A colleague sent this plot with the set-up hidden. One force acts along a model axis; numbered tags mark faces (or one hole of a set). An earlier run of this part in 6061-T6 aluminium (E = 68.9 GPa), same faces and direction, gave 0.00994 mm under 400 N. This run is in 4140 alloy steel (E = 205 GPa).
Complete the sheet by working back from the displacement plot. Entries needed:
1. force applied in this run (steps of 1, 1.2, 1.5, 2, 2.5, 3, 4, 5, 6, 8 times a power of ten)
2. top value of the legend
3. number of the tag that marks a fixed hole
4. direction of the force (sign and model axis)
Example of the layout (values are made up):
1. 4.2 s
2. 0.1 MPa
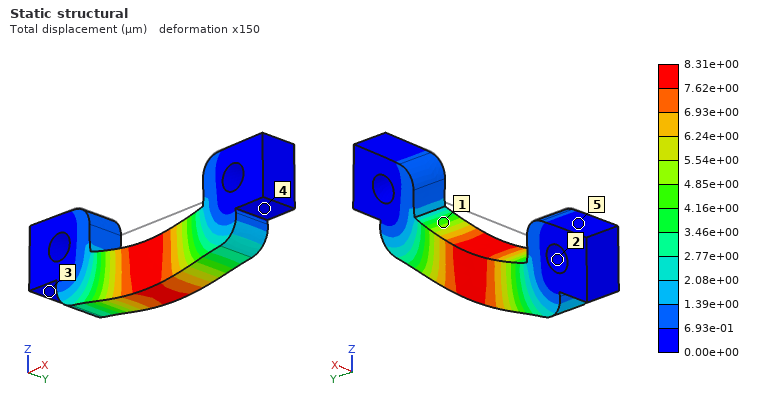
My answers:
1. 1 kN
2. 8.31e+00 µm
3. 2
4. -Z
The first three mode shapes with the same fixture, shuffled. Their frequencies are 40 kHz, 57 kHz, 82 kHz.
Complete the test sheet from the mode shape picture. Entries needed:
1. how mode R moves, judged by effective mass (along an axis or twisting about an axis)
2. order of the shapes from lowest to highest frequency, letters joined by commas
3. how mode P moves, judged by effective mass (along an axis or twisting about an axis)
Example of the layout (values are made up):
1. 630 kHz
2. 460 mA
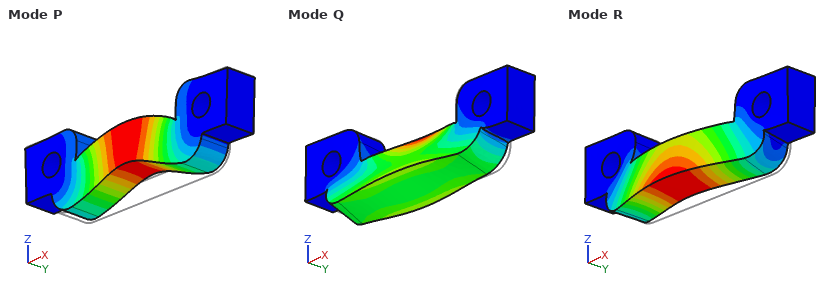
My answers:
1. along Y
2. R, P, Q
3. along Z
